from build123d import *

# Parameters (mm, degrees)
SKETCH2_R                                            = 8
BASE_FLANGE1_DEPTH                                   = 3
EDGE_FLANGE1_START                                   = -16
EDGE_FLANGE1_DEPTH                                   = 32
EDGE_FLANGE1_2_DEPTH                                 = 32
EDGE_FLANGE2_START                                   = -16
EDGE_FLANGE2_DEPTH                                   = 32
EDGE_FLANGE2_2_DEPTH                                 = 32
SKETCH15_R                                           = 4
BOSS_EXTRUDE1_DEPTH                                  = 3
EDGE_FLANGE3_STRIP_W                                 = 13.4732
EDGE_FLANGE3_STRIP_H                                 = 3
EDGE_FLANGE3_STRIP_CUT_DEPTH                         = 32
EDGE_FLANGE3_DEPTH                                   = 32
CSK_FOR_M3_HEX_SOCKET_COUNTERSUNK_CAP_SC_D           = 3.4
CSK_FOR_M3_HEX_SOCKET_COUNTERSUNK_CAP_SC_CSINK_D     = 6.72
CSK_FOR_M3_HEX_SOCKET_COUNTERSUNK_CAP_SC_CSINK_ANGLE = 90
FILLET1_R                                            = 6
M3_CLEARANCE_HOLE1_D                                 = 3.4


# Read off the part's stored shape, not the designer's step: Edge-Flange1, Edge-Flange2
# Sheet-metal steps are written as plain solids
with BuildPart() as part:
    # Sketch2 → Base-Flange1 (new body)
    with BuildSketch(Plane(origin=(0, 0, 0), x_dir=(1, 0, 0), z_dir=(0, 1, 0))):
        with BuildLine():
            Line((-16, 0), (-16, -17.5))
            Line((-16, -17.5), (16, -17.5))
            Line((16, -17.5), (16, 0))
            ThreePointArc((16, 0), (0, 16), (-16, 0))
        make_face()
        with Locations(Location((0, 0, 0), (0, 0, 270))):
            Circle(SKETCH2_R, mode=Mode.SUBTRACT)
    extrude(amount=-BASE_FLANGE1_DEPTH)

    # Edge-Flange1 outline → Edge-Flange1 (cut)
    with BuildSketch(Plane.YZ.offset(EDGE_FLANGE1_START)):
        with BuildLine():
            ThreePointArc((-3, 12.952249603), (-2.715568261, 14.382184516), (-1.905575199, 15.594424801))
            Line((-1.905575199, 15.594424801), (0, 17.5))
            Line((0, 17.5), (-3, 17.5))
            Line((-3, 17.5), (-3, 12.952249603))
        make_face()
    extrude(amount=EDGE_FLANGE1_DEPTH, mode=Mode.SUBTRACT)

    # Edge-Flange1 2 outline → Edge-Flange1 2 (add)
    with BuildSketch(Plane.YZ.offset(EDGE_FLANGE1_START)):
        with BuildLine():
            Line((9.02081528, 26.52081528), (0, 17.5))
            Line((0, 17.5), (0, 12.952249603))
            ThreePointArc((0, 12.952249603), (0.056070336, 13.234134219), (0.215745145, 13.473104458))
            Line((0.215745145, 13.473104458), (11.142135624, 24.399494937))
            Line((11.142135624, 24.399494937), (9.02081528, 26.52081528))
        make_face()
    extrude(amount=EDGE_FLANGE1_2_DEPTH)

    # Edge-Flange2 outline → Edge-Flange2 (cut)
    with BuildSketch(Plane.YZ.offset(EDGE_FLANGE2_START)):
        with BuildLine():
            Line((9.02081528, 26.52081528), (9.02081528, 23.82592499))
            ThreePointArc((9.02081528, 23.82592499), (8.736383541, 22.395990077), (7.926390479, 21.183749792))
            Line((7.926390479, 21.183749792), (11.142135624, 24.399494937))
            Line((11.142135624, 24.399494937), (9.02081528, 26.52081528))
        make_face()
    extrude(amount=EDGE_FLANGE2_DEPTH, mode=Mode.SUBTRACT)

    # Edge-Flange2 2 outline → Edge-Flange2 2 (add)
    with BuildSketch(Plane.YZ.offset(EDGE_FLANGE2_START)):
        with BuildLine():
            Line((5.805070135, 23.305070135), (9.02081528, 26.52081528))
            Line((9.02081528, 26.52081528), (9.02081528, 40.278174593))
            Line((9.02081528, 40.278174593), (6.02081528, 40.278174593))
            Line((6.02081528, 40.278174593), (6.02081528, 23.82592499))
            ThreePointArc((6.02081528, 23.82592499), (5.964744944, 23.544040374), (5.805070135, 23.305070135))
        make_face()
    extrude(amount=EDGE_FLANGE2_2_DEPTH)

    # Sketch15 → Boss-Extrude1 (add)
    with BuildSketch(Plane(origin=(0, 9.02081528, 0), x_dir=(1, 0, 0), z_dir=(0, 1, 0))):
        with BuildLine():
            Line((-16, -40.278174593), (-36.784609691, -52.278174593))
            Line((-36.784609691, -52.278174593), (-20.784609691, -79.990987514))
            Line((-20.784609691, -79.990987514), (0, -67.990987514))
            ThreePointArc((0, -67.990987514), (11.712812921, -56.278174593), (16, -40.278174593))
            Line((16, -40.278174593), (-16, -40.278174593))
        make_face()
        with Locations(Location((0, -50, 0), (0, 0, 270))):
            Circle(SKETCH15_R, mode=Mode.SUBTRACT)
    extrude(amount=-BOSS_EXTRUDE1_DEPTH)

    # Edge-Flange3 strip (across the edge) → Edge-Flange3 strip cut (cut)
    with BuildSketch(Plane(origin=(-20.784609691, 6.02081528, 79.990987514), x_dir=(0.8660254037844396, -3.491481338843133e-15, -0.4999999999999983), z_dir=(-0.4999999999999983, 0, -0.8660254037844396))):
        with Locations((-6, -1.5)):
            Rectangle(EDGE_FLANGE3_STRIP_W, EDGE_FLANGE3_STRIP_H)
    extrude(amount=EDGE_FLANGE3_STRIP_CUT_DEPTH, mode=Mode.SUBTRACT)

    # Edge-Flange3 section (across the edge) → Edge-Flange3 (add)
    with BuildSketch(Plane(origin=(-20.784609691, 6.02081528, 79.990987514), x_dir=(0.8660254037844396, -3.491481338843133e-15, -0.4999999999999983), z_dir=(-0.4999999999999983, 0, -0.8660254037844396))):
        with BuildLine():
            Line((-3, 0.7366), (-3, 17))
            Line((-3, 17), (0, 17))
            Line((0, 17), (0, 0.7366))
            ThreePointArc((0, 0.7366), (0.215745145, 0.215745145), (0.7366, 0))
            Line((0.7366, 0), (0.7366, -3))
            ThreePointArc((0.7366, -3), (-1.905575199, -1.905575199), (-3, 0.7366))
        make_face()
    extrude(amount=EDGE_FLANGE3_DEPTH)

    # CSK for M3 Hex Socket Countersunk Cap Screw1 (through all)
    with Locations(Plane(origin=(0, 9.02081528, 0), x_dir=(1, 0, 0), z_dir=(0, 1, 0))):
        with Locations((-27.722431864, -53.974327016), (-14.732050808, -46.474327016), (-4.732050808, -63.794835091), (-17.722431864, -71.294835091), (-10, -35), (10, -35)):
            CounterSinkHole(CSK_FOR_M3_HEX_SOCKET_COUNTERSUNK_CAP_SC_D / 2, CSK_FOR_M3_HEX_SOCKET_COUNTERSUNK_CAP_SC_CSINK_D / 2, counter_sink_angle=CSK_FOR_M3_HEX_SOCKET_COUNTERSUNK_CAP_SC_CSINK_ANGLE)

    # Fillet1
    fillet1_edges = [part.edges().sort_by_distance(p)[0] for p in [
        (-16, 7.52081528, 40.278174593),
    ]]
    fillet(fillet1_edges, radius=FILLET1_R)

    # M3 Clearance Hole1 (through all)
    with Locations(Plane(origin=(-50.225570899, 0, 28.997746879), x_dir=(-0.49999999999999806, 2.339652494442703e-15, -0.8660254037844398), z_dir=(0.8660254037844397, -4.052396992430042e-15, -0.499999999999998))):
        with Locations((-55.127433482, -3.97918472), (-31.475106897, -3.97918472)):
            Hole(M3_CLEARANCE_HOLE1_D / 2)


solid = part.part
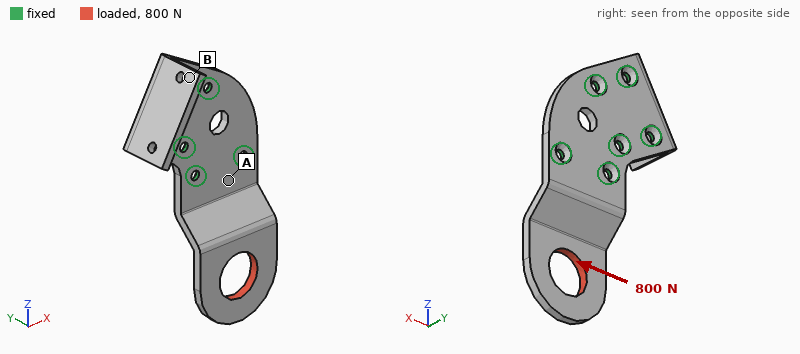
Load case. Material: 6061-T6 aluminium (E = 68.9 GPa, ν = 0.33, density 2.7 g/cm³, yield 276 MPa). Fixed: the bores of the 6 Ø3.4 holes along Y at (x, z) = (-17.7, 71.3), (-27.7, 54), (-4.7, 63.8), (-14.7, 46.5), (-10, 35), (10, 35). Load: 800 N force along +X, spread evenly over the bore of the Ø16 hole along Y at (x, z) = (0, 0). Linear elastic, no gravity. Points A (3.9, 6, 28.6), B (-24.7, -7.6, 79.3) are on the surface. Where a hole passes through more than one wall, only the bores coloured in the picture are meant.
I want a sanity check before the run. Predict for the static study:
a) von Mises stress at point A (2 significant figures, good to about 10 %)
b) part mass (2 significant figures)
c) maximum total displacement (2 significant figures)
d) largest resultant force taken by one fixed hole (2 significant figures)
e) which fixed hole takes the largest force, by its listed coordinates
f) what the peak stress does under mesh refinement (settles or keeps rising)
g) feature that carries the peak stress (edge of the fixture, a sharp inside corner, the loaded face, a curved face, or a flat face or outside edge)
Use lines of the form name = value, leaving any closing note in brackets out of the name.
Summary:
von Mises stress at point A = 64 MPa
part mass = 27 g
maximum total displacement = 0.21 mm
largest resultant force taken by one fixed hole = 1.2 kN
which fixed hole takes the largest force, by its listed coordinates = (10, 35)
what the peak stress does under mesh refinement = keeps rising
feature that carries the peak stress = edge of the fixture
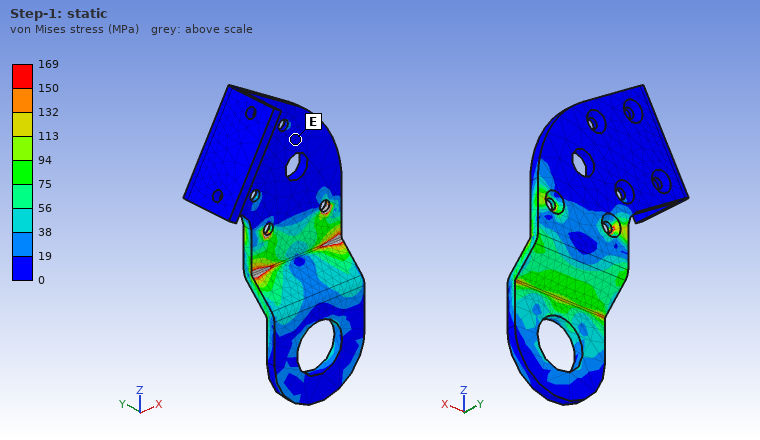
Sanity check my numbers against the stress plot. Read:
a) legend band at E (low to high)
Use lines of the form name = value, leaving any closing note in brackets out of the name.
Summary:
legend band at E = 0 to 19 MPa
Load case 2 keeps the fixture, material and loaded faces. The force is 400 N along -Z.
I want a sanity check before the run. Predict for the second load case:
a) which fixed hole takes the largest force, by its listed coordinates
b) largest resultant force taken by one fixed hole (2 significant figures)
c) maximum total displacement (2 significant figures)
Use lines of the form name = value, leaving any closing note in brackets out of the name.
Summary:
which fixed hole takes the largest force, by its listed coordinates = (-10, 35)
largest resultant force taken by one fixed hole = 330 N
maximum total displacement = 0.62 mm
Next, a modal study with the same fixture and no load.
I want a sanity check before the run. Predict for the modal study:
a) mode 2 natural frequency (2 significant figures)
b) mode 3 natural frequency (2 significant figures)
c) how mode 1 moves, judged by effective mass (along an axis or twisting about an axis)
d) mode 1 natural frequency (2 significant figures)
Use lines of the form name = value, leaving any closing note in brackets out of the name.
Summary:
mode 2 natural frequency = 3400 Hz
mode 3 natural frequency = 3900 Hz
how mode 1 moves, judged by effective mass = along Y
mode 1 natural frequency = 1000 Hz
